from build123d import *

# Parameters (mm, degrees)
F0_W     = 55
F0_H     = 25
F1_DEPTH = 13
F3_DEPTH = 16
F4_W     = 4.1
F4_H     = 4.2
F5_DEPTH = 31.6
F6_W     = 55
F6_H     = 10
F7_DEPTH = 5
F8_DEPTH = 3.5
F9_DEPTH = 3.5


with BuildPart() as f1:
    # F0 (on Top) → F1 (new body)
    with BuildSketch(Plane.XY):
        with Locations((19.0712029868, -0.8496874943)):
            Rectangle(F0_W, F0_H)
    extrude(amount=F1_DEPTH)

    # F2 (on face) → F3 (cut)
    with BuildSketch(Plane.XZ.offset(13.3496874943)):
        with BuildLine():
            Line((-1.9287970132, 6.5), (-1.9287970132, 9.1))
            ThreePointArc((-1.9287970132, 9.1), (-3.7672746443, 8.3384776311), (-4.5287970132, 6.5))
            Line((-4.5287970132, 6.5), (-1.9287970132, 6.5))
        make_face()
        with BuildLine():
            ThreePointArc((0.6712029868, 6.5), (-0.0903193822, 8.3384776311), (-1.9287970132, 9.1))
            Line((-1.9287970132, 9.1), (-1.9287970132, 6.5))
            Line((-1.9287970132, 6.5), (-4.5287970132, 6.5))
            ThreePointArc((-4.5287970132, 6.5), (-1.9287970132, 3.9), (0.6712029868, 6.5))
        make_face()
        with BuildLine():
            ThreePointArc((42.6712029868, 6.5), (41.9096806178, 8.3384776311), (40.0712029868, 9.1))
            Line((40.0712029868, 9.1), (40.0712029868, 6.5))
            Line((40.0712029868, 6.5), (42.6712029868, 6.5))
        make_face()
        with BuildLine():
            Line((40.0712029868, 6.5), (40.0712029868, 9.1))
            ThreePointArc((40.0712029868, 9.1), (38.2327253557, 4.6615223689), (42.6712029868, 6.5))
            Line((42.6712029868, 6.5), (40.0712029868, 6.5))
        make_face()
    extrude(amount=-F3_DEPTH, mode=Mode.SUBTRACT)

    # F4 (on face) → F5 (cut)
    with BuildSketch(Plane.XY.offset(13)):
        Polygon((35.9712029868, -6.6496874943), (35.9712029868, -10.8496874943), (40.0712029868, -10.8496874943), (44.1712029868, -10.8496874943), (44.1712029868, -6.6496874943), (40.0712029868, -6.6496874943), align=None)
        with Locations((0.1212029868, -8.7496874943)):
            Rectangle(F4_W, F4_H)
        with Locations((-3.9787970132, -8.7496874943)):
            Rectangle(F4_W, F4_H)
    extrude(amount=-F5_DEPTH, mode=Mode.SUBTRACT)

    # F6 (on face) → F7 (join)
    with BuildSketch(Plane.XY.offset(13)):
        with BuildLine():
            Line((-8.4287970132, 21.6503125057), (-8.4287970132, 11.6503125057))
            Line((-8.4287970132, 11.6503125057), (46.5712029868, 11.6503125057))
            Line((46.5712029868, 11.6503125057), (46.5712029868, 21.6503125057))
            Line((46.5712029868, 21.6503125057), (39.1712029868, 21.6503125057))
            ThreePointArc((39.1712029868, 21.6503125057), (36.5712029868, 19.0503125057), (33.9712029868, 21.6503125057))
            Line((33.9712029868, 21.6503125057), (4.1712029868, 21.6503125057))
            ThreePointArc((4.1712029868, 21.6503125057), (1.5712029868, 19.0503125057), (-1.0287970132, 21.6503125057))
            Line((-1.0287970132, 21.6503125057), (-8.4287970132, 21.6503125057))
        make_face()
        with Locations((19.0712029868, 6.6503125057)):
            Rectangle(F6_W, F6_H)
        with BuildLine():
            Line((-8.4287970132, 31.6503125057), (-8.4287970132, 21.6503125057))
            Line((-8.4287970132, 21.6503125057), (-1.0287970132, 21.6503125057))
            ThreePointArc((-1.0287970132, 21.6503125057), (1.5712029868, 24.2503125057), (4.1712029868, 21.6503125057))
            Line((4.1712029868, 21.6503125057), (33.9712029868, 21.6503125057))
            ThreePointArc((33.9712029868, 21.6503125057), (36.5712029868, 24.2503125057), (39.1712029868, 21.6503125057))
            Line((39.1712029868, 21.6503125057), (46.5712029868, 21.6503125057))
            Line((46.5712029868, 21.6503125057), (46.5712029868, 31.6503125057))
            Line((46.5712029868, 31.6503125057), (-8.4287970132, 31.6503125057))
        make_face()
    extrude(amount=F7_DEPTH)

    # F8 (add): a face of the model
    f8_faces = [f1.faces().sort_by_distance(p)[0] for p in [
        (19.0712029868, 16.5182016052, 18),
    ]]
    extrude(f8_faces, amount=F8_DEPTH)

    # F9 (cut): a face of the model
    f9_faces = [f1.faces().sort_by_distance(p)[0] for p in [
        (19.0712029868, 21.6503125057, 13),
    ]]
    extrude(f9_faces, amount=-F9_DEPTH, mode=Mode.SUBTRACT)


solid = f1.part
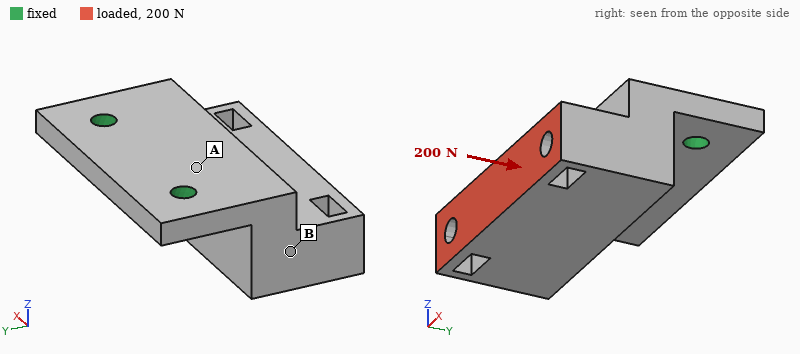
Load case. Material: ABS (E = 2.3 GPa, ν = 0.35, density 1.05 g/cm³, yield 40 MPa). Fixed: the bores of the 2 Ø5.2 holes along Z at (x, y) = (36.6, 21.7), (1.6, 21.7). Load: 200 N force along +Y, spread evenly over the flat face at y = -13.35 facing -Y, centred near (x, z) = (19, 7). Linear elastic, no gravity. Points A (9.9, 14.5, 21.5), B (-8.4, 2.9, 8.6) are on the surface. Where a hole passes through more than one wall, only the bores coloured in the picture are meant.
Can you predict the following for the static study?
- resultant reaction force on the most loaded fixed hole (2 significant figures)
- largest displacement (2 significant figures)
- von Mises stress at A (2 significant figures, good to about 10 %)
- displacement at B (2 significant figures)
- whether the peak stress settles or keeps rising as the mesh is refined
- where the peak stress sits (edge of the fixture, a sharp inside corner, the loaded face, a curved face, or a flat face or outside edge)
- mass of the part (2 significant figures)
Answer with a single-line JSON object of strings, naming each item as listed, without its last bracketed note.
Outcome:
{"resultant reaction force on the most loaded fixed hole": "100 N", "largest displacement": "0.83 mm", "von Mises stress at A": "8.2 MPa", "displacement at B": "0.38 mm", "whether the peak stress settles or keeps rising as the mesh is refined": "keeps rising", "where the peak stress sits": "edge of the fixture", "mass of the part": "28 g"}
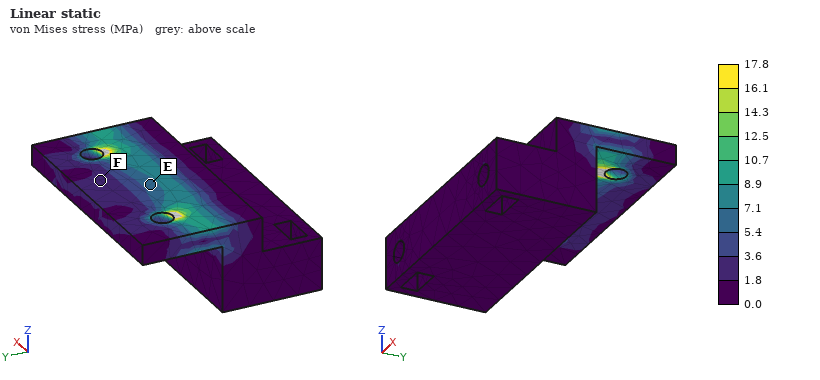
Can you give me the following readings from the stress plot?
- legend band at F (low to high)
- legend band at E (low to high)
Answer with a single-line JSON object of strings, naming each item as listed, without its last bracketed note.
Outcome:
{"legend band at F": "1.8 to 3.6 MPa", "legend band at E": "5.4 to 7.1 MPa"}
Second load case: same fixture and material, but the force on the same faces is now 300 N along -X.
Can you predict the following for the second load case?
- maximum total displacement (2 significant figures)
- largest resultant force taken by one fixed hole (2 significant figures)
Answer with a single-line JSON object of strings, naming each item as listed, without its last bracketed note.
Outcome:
{"maximum total displacement": "0.14 mm", "largest resultant force taken by one fixed hole": "330 N"}
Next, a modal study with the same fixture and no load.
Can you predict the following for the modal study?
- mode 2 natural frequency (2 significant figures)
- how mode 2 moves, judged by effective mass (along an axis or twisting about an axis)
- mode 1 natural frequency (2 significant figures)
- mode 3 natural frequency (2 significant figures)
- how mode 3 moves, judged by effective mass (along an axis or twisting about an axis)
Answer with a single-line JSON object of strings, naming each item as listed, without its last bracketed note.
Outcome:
{"mode 2 natural frequency": "1800 Hz", "how mode 2 moves, judged by effective mass": "along X", "mode 1 natural frequency": "540 Hz", "mode 3 natural frequency": "2700 Hz", "how mode 3 moves, judged by effective mass": "along X"}
